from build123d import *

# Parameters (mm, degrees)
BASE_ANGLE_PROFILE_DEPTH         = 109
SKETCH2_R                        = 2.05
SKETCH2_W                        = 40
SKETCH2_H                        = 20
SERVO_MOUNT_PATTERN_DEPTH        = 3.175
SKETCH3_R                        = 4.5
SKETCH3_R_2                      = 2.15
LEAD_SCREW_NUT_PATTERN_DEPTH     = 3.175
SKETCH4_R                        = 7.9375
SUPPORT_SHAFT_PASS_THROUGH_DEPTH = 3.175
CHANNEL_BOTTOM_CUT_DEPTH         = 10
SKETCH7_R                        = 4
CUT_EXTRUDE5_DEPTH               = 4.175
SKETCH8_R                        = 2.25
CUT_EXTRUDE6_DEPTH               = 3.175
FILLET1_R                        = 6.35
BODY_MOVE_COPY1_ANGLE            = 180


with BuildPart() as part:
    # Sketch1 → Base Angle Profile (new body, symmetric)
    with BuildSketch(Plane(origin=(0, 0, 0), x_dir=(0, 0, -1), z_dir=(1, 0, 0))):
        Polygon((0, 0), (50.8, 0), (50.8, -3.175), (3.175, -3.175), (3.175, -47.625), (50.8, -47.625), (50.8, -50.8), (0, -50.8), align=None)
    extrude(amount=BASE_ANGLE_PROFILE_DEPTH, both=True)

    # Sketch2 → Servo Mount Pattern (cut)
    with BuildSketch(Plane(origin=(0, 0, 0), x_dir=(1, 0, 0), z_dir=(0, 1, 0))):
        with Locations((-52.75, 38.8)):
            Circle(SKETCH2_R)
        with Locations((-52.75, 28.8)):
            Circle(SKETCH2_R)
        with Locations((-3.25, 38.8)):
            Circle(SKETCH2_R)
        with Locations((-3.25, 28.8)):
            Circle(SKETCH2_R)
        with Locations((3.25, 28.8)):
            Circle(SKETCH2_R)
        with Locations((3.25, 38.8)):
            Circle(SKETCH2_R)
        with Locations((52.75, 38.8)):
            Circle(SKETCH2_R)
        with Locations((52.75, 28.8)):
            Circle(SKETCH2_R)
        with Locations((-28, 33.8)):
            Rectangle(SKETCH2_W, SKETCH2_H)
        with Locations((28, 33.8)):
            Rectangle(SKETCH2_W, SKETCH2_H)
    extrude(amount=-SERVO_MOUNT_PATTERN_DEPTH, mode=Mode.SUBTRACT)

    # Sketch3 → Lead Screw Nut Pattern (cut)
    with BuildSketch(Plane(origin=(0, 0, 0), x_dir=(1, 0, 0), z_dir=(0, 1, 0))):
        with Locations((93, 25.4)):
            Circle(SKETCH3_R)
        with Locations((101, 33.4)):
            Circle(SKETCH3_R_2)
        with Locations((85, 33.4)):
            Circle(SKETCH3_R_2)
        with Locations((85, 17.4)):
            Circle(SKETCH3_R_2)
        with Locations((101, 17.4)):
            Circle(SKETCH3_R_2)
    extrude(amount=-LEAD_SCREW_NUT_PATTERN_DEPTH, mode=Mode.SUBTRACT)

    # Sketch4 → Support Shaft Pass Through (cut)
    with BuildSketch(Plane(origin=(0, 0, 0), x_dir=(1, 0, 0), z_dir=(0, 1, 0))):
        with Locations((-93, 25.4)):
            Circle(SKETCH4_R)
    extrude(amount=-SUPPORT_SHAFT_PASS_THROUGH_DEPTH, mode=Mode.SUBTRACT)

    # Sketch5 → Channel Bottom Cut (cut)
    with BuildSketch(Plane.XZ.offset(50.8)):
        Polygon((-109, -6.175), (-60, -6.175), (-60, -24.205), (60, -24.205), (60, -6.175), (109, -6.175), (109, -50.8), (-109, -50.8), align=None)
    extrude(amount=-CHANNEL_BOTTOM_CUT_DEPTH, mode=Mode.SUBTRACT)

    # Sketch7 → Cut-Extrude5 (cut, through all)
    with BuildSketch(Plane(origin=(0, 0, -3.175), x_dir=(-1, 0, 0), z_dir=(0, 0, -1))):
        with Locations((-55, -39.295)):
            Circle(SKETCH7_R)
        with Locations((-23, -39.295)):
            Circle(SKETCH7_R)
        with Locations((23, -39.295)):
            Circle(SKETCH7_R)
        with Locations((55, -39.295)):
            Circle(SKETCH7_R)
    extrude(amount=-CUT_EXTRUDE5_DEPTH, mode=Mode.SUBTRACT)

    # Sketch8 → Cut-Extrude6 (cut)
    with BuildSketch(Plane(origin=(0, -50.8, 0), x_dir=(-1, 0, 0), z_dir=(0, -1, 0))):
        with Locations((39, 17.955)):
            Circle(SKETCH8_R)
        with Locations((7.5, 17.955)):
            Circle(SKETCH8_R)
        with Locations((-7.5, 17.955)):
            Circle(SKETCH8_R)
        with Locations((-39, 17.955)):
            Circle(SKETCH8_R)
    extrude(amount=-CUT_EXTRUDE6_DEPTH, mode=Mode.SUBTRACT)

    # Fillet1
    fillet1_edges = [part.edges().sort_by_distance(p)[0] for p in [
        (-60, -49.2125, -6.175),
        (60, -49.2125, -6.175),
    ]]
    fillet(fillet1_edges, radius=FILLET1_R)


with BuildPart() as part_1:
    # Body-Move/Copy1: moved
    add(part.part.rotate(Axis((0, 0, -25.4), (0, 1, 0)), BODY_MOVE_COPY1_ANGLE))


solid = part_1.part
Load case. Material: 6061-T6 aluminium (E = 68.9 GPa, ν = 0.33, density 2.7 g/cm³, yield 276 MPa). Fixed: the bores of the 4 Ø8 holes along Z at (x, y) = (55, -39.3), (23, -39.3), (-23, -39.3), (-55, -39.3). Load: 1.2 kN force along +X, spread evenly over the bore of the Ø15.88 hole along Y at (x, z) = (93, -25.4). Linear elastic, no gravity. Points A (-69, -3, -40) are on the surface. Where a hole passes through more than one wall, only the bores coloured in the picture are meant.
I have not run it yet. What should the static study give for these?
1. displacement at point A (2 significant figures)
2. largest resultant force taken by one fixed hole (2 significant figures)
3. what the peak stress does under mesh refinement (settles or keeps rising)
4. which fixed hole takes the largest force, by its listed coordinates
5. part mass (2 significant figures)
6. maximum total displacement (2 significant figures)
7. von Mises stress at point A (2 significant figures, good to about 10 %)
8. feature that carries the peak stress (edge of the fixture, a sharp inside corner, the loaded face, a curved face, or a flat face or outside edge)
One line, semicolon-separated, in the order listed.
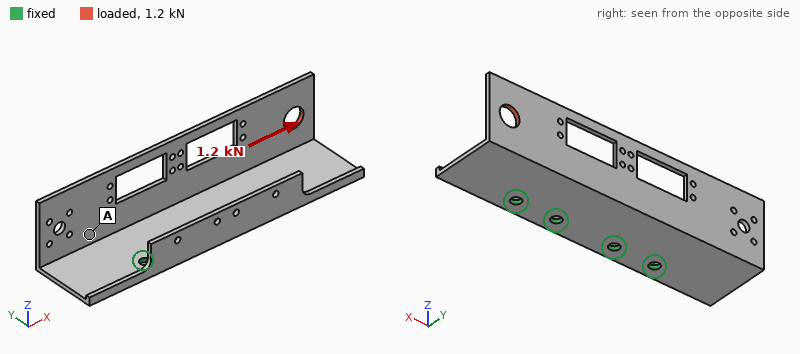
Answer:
0.26 mm; 540 N; keeps rising; (55, -39.3); 190 g; 0.64 mm; 10 MPa; edge of the fixture
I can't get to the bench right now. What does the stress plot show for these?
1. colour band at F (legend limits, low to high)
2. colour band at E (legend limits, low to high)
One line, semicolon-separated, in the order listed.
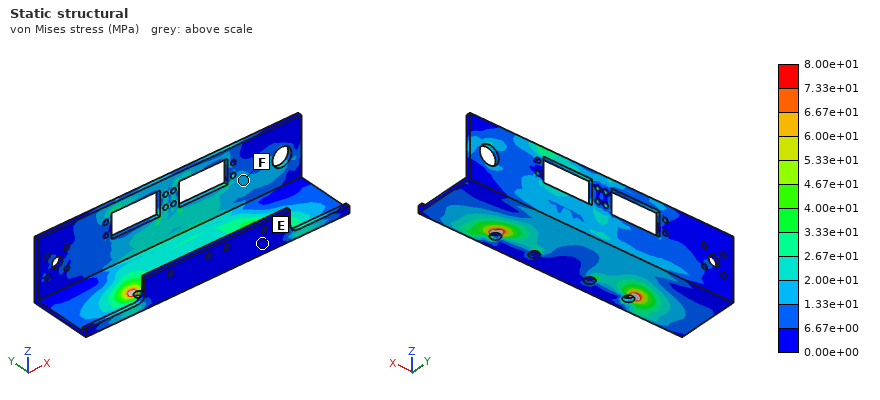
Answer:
1.33e+01 to 2.00e+01 MPa; 0.00e+00 to 6.67e+00 MPa
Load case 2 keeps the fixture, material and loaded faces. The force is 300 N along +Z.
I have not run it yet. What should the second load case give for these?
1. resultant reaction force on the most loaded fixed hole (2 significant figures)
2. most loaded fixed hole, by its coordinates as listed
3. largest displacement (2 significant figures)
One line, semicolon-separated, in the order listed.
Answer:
320 N; (55, -39.3); 0.90 mm
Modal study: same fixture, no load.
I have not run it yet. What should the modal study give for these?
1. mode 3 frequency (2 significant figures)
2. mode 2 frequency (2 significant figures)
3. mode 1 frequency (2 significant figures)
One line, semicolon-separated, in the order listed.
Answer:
1000 Hz; 520 Hz; 500 Hz
